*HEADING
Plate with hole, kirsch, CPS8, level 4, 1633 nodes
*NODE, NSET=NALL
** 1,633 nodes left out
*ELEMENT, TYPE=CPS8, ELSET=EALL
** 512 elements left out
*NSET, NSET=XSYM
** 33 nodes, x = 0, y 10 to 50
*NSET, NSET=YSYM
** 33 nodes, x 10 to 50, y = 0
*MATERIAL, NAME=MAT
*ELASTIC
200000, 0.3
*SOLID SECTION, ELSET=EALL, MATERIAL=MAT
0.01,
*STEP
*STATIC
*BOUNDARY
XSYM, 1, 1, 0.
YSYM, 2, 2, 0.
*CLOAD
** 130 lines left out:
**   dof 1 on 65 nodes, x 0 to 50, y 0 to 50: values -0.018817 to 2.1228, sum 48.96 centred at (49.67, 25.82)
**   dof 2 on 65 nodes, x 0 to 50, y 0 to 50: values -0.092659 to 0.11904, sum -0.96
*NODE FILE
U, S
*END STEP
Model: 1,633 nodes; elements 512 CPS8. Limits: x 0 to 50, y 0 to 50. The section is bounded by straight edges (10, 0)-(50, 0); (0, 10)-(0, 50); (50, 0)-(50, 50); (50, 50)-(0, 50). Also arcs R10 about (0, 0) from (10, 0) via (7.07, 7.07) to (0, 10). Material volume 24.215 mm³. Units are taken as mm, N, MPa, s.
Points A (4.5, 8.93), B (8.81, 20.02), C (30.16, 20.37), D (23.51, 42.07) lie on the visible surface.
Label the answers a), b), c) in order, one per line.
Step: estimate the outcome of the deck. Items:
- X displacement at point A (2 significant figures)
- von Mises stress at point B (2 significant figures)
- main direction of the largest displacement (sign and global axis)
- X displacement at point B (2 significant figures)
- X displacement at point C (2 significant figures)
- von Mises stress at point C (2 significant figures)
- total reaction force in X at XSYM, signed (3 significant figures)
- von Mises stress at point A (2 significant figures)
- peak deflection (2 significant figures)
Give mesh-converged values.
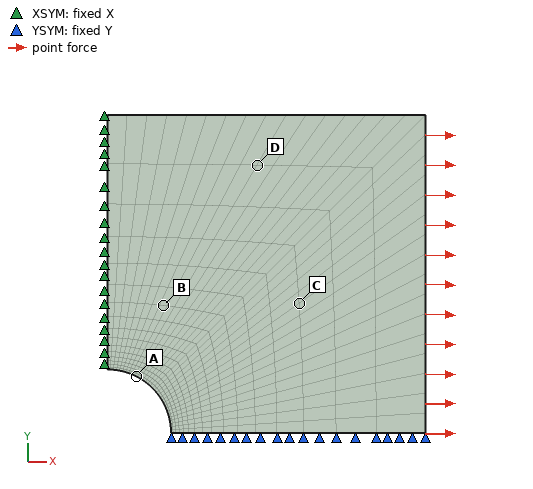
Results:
a) 0.0067 mm
b) 120 MPa
c) +X
d) 0.0051 mm
e) 0.017 mm
f) 100 MPa
g) -49.0 N
h) 220 MPa
i) 0.028 mm
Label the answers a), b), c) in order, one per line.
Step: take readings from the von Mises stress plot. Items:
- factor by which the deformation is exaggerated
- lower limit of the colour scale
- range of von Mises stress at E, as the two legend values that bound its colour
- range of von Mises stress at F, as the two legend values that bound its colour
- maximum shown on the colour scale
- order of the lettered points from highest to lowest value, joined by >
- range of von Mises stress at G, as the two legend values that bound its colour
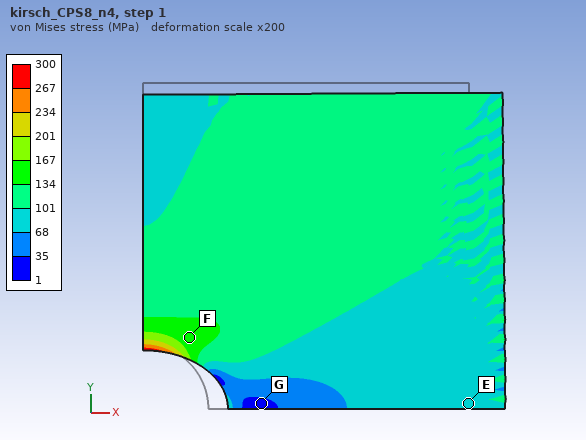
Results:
a) 200
b) 1 MPa
c) 68 to 101 MPa
d) 134 to 167 MPa
e) 300 MPa
f) F > E > G
g) 1 to 35 MPa
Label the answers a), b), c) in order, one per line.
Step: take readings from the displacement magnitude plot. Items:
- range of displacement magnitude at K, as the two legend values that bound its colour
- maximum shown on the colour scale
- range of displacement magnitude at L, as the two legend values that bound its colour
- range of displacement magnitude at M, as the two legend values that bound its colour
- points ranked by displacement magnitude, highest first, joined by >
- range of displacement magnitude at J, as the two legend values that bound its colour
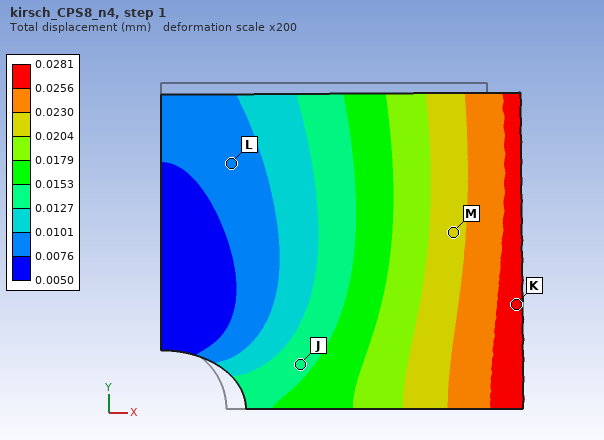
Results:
a) 0.0256 to 0.0281 mm
b) 0.0281 mm
c) 0.0076 to 0.0101 mm
d) 0.0204 to 0.0230 mm
e) K > M > J > L
f) 0.0127 to 0.0153 mm
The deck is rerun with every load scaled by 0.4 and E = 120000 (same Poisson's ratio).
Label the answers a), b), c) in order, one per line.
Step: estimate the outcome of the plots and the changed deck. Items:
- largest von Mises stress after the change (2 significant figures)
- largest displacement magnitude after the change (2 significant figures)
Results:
a) 120 MPa
b) 0.019 mm
